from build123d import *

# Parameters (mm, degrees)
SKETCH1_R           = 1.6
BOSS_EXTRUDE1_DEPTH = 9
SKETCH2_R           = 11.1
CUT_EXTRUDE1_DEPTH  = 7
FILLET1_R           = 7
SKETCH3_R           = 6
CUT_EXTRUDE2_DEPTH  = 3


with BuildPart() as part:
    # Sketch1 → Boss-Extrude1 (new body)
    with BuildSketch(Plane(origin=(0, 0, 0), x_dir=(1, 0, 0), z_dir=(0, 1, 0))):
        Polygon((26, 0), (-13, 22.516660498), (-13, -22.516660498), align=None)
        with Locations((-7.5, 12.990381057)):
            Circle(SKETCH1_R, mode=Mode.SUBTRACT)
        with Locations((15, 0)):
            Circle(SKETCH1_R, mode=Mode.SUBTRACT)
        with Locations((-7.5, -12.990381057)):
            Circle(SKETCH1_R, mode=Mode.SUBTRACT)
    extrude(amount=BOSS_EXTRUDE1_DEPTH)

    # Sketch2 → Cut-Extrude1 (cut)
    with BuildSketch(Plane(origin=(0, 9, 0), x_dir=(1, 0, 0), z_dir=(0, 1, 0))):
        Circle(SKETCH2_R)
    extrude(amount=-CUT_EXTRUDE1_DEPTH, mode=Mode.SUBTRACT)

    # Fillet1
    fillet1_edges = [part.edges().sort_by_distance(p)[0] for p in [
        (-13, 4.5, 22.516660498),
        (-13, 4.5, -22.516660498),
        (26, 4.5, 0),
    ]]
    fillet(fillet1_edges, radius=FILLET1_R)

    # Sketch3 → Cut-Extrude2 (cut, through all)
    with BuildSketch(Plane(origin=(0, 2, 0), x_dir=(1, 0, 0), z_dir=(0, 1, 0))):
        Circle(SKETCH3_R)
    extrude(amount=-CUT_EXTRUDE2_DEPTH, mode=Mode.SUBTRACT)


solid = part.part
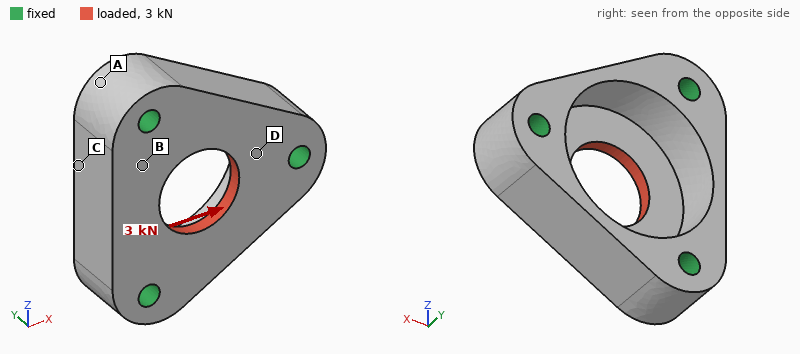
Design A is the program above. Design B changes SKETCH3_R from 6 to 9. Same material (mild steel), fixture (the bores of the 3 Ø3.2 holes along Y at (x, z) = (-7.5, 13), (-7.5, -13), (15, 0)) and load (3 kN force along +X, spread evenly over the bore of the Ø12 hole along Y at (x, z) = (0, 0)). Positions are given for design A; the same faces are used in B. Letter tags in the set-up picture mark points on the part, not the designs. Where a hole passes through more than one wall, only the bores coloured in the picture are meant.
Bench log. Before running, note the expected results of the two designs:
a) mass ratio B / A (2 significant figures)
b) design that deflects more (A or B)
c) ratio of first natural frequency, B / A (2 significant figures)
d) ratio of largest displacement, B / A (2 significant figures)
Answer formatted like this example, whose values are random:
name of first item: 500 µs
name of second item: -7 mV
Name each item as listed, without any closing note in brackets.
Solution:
mass ratio B / A: 0.93
design that deflects more: B
ratio of first natural frequency, B / A: 1.1
ratio of largest displacement, B / A: 1.1
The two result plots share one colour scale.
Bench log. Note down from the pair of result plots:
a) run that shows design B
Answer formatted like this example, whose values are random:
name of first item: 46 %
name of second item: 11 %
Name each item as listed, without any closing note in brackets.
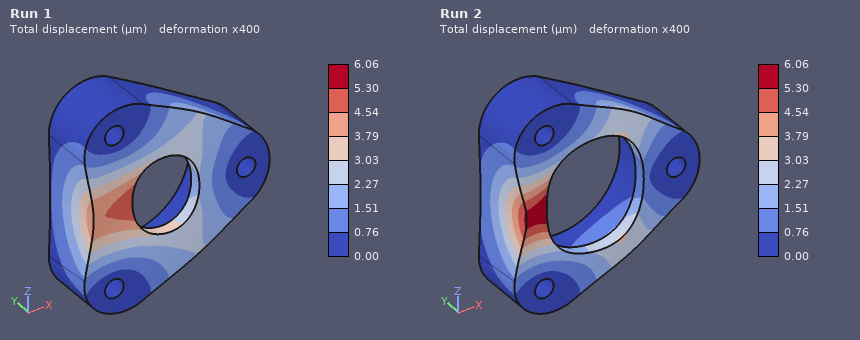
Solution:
run that shows design B: Run 2
